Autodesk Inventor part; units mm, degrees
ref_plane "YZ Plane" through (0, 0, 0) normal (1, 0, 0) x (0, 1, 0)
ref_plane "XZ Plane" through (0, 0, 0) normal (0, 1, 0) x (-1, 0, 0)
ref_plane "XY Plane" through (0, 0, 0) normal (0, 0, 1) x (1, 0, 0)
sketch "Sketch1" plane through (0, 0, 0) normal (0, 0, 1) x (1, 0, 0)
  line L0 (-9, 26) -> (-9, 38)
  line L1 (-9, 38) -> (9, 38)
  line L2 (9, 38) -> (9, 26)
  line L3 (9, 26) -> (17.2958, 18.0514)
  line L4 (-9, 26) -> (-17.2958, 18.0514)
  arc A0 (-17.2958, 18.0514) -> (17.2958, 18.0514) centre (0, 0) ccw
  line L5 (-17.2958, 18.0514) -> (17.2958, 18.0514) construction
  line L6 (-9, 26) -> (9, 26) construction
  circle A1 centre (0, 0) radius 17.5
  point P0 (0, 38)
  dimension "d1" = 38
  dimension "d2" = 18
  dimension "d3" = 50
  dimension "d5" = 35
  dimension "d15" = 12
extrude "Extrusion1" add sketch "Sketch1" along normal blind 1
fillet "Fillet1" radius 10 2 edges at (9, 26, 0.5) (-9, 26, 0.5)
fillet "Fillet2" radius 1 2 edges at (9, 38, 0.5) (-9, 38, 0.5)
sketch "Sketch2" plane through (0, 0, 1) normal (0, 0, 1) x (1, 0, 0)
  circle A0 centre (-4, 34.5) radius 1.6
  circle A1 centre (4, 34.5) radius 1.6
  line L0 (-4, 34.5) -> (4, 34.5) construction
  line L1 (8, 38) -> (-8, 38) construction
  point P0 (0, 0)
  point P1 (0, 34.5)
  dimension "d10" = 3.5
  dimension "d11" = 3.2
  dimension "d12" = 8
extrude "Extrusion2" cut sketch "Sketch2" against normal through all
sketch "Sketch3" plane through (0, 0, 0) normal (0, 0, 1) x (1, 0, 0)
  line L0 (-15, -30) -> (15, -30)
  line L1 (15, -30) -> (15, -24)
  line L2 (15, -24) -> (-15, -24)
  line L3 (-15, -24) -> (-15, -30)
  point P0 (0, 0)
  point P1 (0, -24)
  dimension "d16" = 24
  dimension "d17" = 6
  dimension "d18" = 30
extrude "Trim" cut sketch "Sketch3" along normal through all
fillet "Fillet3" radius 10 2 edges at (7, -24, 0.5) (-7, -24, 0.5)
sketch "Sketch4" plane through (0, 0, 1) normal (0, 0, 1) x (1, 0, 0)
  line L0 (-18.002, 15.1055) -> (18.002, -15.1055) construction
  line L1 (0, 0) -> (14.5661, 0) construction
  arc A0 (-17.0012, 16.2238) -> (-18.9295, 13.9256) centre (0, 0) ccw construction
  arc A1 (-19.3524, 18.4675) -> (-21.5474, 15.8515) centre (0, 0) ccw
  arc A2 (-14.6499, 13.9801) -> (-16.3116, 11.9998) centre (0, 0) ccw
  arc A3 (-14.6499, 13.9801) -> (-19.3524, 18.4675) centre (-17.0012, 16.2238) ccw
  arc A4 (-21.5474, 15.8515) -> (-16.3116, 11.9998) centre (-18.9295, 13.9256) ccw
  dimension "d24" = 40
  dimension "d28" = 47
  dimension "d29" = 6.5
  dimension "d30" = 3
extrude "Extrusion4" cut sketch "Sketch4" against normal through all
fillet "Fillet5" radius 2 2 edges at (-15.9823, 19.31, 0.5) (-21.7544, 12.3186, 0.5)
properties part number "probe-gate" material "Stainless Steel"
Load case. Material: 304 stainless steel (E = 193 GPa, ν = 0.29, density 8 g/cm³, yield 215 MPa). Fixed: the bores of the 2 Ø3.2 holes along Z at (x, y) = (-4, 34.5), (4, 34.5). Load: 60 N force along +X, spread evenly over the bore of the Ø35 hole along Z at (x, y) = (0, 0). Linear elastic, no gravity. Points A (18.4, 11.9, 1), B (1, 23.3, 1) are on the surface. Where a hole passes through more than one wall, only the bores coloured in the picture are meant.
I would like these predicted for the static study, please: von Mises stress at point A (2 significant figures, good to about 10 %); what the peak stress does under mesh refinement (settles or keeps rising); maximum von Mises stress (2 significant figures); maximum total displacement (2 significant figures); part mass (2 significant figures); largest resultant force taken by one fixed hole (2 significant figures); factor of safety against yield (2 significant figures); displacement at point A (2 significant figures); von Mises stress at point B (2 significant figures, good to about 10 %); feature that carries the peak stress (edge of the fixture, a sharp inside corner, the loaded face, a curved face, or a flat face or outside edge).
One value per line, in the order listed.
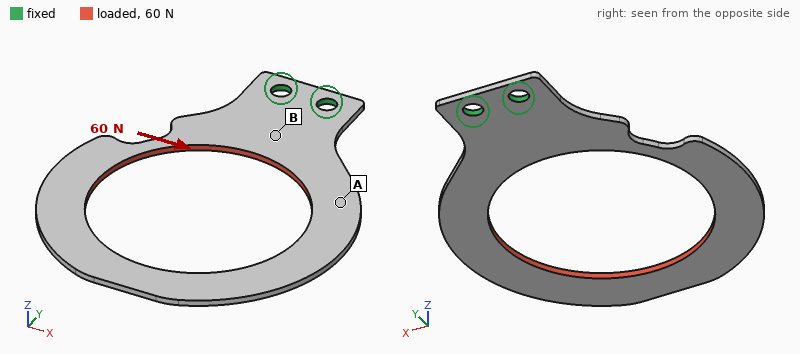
11 MPa
settles
90 MPa
53 µm
9.6 g
200 N
2.4
16 µm
23 MPa
a curved face
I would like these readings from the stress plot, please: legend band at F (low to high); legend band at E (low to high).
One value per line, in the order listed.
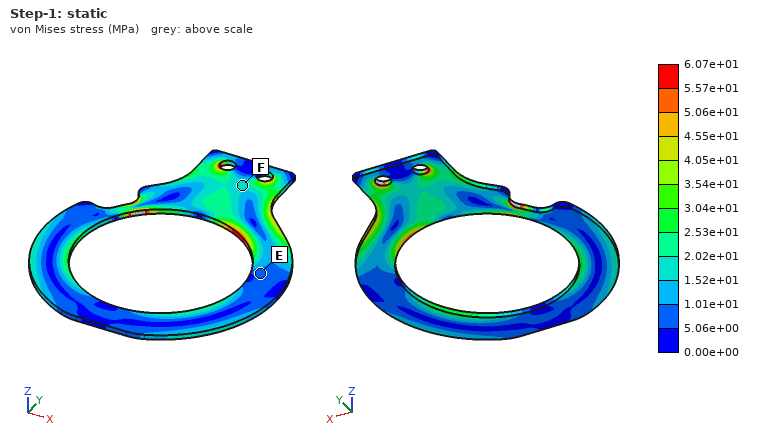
1.52e+01 to 2.02e+01 MPa
5.06e+00 to 1.01e+01 MPa
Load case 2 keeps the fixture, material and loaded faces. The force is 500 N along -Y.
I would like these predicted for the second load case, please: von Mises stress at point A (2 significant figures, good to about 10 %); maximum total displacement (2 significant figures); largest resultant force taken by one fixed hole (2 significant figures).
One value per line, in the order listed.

26 MPa
47 µm
250 N
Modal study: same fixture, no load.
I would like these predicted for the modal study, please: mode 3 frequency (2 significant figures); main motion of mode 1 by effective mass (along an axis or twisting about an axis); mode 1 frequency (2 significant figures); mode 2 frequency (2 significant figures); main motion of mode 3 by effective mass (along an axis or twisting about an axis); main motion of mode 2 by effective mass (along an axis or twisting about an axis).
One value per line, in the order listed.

1100 Hz
along Z
200 Hz
460 Hz
along Z
twisting about Y
